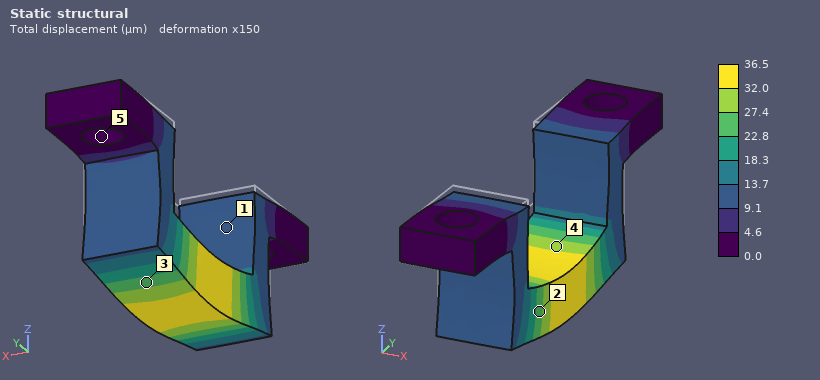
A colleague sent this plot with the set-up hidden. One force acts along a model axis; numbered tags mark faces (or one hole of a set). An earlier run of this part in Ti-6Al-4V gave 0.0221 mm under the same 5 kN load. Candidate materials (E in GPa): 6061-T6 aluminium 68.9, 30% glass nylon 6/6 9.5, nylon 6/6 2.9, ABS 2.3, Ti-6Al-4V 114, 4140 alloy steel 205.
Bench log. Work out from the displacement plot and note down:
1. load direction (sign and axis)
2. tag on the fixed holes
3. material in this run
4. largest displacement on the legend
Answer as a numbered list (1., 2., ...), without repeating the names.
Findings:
1. -Z
2. 5
3. 6061-T6 aluminium
4. 36.5 µm
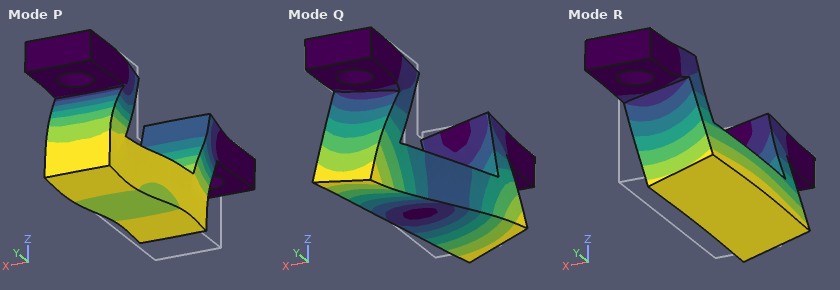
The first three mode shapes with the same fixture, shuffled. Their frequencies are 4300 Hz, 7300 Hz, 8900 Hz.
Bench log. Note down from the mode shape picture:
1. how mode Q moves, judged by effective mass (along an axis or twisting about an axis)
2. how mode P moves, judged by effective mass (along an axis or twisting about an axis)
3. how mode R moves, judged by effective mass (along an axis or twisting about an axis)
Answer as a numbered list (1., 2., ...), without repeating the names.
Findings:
1. twisting about Z
2. along Y
3. along X
